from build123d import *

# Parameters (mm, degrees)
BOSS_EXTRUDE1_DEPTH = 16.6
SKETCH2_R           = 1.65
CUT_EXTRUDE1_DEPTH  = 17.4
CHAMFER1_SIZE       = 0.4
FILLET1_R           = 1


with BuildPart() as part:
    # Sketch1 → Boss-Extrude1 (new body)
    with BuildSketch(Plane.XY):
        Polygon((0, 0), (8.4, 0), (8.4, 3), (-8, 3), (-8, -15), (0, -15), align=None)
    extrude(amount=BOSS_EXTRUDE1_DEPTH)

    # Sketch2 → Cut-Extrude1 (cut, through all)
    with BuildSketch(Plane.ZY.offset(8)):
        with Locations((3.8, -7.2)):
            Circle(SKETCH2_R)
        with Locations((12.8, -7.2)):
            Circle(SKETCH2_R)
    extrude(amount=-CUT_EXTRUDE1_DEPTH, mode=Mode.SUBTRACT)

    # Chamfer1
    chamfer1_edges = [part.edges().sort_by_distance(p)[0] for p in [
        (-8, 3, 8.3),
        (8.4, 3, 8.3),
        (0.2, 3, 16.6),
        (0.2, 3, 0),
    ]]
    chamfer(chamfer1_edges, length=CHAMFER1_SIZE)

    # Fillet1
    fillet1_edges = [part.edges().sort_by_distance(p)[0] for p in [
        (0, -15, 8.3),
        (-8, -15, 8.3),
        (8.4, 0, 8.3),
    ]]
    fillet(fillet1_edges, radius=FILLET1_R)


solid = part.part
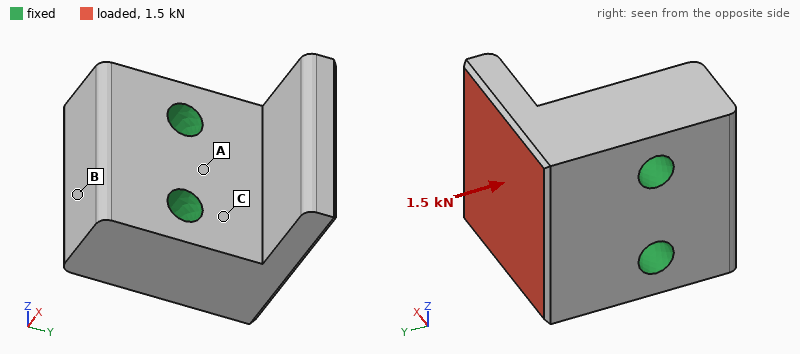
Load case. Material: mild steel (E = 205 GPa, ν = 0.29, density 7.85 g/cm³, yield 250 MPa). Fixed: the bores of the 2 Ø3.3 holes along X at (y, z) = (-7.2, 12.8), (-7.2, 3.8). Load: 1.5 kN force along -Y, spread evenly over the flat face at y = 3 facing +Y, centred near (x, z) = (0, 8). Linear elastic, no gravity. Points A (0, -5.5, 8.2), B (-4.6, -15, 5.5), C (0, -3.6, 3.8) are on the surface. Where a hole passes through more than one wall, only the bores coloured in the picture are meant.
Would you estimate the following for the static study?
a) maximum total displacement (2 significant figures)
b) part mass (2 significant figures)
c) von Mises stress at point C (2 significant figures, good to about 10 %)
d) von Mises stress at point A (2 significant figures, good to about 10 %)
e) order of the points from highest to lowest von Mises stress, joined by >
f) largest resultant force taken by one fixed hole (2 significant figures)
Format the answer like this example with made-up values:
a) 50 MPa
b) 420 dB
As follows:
a) 19 µm
b) 21 g
c) 56 MPa
d) 25 MPa
e) C > A > B
f) 770 N
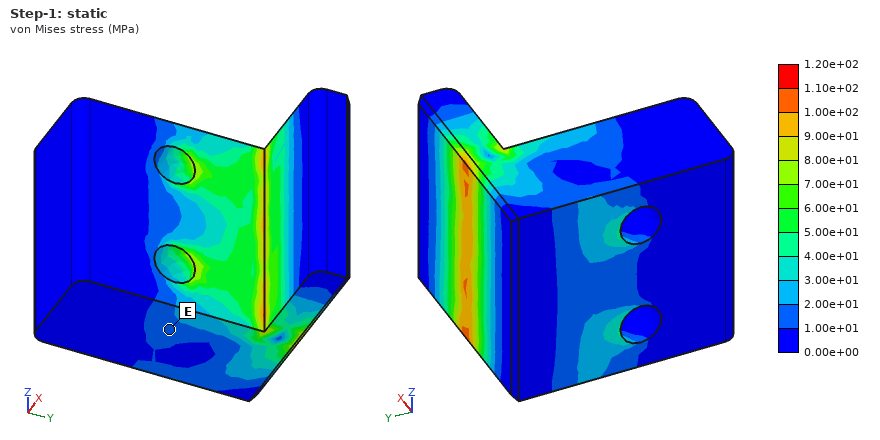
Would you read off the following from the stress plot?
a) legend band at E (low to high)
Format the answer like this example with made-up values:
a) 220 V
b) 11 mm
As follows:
a) 1.00e+01 to 2.00e+01 MPa
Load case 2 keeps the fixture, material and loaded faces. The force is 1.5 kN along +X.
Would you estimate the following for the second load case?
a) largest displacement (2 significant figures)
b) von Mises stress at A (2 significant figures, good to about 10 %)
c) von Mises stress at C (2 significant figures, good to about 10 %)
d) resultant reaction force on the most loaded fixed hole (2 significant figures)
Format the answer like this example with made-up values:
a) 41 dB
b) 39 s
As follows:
a) 14 µm
b) 38 MPa
c) 70 MPa
d) 750 N
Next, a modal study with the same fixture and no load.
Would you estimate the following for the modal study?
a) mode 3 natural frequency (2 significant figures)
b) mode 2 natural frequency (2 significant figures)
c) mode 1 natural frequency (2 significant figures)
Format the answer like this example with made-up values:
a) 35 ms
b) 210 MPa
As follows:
a) 37 kHz
b) 33 kHz
c) 21 kHz
